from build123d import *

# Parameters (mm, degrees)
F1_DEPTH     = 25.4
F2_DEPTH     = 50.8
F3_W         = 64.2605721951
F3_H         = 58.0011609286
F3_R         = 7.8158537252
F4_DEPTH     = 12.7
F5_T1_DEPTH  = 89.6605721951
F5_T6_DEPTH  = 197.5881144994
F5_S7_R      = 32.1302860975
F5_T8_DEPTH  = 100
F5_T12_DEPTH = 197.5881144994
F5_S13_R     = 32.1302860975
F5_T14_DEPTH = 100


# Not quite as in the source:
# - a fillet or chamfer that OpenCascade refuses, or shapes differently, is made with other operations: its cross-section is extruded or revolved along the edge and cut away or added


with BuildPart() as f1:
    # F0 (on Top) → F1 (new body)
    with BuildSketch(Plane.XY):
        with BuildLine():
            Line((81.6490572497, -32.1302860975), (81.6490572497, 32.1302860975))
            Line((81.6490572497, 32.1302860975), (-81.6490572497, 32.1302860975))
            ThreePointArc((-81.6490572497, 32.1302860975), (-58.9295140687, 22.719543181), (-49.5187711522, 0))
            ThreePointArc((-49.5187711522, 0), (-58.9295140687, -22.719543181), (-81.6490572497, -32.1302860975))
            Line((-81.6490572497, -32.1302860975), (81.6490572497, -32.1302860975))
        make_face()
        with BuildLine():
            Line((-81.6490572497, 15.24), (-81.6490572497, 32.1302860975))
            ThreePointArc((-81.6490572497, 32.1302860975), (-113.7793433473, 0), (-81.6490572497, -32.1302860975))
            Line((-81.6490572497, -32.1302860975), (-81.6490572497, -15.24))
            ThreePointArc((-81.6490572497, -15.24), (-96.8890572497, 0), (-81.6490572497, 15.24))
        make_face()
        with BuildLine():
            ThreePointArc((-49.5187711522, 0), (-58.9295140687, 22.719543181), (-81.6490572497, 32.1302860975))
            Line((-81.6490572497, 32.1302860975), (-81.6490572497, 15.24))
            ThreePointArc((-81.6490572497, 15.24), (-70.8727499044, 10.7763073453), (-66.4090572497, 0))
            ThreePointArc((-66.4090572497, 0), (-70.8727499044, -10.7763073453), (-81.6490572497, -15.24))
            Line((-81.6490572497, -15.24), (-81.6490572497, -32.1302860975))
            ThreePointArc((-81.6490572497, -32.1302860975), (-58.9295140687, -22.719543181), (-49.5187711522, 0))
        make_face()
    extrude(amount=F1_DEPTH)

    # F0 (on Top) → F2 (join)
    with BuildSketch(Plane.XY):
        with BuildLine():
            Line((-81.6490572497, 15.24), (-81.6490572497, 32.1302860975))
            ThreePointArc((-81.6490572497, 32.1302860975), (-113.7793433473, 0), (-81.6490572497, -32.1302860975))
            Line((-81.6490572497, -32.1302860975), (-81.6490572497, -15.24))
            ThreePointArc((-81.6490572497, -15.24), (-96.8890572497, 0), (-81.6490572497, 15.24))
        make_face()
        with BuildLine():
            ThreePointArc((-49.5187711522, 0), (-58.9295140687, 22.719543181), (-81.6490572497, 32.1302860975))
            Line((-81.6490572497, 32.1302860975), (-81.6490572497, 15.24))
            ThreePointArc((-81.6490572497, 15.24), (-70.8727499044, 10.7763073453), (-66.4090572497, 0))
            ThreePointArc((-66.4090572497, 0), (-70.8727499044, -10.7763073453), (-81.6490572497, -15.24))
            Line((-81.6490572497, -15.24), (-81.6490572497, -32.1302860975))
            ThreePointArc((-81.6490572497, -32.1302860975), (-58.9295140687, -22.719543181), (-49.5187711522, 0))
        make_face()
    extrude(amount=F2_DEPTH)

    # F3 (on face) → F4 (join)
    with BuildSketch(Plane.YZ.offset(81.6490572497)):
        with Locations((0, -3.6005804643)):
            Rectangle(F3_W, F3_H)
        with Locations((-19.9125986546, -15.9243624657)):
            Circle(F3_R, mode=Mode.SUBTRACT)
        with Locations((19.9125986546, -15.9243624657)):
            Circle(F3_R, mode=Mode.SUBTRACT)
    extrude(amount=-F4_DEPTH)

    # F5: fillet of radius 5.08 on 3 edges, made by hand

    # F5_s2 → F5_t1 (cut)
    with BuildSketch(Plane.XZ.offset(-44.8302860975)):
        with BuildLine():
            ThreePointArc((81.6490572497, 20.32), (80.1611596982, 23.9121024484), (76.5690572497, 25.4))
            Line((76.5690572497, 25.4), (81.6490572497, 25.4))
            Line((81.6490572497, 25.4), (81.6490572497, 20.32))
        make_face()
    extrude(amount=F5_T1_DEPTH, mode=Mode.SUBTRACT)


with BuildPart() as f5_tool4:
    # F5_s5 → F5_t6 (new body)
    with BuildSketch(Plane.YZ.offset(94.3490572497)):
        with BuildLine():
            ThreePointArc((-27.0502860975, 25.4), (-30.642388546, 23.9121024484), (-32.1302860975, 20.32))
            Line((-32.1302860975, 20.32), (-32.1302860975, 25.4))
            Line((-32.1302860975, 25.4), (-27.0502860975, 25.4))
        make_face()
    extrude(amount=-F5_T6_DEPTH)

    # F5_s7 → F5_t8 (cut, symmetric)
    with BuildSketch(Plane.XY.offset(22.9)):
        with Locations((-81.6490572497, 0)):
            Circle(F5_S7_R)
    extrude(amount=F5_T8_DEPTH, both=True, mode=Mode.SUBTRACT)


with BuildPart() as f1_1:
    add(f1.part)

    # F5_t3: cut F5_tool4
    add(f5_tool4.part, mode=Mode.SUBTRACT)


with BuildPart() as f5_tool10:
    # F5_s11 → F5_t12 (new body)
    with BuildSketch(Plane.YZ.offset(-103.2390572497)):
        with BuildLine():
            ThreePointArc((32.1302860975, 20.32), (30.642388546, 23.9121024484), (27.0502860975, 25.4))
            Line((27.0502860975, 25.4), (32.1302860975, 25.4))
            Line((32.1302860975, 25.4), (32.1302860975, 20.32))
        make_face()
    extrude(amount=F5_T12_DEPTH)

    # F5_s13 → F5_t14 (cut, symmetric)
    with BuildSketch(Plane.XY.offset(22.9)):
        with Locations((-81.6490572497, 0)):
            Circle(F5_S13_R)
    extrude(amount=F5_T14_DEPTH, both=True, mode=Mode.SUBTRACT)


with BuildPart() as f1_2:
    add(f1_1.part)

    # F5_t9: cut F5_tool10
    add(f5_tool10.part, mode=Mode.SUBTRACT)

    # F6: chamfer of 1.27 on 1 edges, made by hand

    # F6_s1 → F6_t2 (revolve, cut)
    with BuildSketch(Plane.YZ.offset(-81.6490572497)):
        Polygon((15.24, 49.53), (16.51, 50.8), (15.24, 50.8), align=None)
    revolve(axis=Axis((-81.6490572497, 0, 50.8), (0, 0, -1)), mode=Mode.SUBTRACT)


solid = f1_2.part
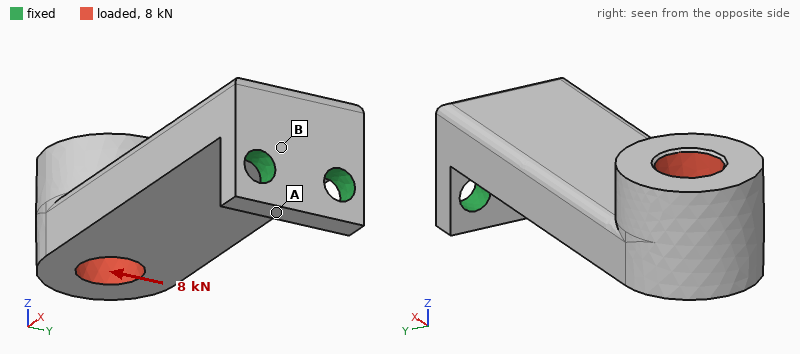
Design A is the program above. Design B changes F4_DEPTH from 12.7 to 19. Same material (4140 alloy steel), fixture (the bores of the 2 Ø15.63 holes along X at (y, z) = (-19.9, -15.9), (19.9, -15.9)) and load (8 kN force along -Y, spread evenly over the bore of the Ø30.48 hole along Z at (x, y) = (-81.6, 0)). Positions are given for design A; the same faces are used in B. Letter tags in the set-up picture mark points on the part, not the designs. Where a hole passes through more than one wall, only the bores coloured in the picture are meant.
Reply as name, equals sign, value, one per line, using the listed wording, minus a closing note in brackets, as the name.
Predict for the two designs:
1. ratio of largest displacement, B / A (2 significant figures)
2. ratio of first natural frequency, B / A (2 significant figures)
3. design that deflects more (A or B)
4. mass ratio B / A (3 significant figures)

ratio of largest displacement, B / A = 0.67
ratio of first natural frequency, B / A = 1.4
design that deflects more = A
mass ratio B / A = 1.03
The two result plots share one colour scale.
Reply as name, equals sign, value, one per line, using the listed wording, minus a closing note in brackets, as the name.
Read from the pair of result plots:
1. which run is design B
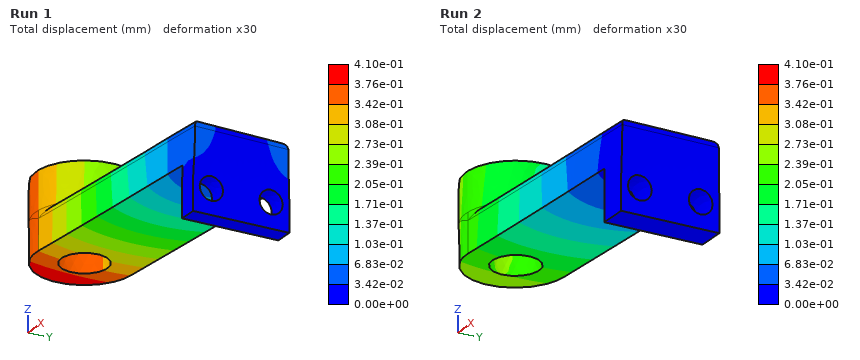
which run is design B = Run 2
